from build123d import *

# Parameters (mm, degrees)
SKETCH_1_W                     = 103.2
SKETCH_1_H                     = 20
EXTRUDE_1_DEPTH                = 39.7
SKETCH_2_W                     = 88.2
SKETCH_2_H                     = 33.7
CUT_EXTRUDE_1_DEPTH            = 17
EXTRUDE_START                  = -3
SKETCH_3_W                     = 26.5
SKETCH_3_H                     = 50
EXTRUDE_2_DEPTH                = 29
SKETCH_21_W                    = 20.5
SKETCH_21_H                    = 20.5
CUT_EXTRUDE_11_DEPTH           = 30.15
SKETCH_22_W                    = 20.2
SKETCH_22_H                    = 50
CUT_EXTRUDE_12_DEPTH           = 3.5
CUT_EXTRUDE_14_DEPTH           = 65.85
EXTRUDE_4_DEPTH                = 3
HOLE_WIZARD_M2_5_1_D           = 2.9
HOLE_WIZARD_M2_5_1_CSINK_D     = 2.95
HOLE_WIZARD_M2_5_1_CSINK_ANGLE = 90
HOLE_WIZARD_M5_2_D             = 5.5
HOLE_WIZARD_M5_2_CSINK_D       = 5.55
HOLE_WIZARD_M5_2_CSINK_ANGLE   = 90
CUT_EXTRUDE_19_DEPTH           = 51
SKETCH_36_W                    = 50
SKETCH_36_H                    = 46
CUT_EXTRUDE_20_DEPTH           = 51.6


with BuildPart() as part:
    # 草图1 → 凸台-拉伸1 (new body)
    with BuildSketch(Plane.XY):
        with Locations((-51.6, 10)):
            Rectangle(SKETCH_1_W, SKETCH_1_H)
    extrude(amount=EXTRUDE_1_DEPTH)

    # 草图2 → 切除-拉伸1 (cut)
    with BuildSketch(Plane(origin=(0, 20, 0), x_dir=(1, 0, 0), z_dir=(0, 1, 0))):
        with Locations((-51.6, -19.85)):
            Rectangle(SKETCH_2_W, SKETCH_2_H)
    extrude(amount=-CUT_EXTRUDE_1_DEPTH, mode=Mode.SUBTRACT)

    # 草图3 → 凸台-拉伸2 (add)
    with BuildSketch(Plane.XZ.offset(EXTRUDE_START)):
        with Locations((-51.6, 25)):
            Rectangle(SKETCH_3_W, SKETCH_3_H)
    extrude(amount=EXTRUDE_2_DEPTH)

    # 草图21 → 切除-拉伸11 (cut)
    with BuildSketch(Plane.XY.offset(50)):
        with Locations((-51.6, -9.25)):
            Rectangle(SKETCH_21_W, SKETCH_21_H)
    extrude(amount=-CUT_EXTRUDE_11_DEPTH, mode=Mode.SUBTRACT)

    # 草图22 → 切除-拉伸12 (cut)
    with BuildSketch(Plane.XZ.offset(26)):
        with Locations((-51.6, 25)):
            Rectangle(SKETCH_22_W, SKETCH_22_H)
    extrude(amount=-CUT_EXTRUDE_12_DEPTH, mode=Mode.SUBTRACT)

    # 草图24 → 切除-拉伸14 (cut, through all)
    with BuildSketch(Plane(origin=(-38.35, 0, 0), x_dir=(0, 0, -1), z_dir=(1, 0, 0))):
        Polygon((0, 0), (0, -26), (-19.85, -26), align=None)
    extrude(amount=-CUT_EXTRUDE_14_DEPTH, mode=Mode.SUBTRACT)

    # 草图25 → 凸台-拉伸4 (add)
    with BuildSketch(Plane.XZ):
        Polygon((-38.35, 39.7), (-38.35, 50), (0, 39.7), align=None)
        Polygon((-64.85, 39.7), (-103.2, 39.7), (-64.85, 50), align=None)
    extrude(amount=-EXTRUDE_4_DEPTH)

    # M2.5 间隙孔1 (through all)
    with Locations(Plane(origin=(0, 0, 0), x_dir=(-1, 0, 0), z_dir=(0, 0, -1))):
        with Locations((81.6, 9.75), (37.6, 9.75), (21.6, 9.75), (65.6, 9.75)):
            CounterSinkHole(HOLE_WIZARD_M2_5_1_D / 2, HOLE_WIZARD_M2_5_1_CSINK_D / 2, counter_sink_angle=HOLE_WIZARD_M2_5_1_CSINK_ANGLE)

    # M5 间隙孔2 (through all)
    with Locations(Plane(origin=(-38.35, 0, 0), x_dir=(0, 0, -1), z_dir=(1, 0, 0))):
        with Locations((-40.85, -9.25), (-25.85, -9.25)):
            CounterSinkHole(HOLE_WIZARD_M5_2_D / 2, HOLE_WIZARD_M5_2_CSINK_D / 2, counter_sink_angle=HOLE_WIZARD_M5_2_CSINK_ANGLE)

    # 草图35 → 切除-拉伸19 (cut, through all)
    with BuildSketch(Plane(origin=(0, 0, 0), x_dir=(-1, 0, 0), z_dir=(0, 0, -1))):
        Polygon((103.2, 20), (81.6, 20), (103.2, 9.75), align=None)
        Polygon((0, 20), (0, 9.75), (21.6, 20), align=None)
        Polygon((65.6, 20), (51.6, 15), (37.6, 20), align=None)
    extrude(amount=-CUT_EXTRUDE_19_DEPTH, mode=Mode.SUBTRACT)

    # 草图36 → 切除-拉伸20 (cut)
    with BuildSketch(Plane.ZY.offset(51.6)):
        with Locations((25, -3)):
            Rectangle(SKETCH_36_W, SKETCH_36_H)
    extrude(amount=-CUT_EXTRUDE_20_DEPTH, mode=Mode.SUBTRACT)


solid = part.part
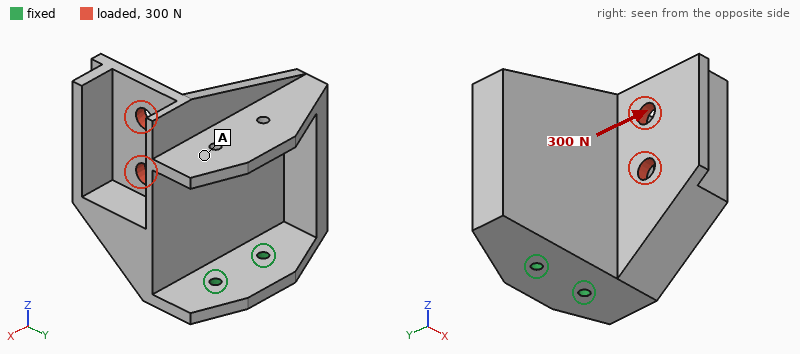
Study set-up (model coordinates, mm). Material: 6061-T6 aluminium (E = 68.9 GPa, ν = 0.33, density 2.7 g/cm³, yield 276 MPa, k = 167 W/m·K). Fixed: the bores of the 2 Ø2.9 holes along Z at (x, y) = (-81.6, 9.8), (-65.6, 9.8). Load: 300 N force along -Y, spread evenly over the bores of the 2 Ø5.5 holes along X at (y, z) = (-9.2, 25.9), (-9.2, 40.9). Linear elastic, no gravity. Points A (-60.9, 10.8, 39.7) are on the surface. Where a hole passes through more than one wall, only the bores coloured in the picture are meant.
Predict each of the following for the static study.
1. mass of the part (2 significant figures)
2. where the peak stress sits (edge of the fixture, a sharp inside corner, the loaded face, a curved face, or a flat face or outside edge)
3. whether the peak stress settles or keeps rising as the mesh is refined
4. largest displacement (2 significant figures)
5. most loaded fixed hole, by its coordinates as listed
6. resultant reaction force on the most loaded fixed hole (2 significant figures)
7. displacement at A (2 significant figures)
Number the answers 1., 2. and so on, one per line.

1. 54 g
2. edge of the fixture
3. keeps rising
4. 0.83 mm
5. (-65.6, 9.8)
6. 310 N
7. 0.56 mm
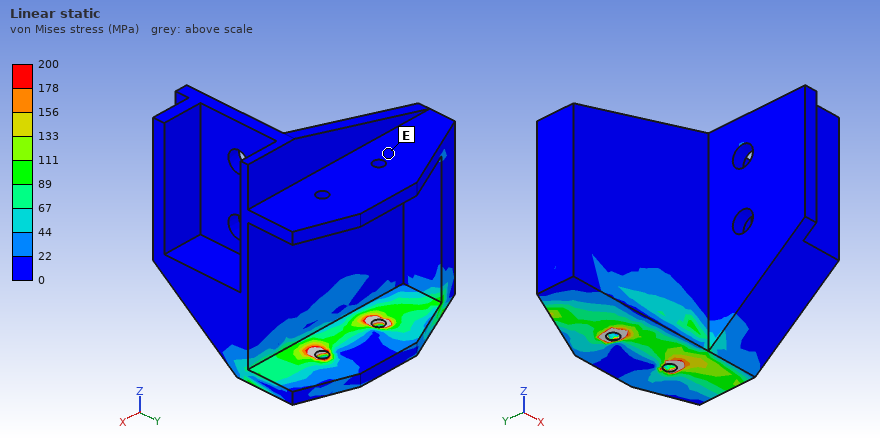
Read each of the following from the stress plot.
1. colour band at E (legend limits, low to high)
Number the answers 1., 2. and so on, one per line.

1. 0 to 22 MPa
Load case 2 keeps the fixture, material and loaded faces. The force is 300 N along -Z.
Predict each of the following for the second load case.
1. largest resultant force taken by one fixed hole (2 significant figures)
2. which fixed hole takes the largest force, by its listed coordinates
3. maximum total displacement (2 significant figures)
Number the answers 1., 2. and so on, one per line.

1. 290 N
2. (-65.6, 9.8)
3. 0.39 mm
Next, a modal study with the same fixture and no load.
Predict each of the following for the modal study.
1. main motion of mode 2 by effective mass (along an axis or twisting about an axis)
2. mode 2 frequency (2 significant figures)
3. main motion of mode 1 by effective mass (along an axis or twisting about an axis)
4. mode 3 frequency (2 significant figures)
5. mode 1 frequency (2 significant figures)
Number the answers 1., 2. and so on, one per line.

1. along X
2. 1600 Hz
3. along Y
4. 2500 Hz
5. 670 Hz
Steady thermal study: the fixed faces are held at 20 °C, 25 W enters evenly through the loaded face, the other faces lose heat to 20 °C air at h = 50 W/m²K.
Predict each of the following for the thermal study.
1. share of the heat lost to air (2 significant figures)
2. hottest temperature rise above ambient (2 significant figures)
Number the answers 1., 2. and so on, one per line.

1. 37 %
2. 33 K
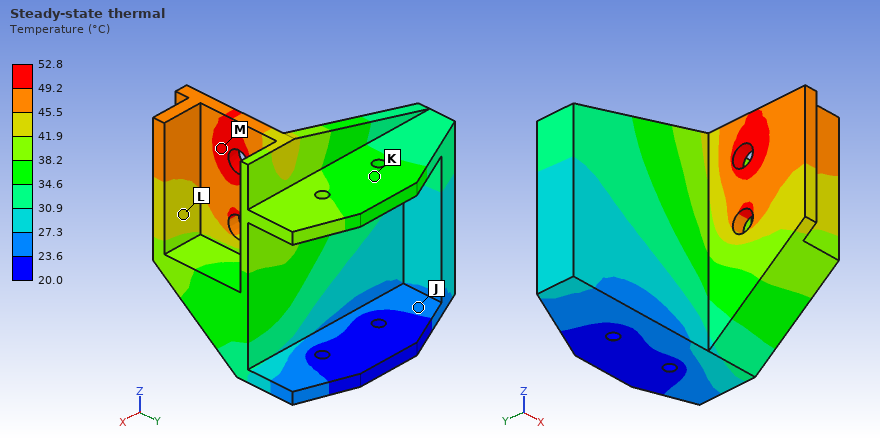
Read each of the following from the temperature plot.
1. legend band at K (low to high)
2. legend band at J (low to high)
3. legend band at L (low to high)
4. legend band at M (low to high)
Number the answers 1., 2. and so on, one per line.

1. 34.6 to 38.2 °C
2. 23.6 to 27.3 °C
3. 41.9 to 45.5 °C
4. 49.2 to 52.8 °C
